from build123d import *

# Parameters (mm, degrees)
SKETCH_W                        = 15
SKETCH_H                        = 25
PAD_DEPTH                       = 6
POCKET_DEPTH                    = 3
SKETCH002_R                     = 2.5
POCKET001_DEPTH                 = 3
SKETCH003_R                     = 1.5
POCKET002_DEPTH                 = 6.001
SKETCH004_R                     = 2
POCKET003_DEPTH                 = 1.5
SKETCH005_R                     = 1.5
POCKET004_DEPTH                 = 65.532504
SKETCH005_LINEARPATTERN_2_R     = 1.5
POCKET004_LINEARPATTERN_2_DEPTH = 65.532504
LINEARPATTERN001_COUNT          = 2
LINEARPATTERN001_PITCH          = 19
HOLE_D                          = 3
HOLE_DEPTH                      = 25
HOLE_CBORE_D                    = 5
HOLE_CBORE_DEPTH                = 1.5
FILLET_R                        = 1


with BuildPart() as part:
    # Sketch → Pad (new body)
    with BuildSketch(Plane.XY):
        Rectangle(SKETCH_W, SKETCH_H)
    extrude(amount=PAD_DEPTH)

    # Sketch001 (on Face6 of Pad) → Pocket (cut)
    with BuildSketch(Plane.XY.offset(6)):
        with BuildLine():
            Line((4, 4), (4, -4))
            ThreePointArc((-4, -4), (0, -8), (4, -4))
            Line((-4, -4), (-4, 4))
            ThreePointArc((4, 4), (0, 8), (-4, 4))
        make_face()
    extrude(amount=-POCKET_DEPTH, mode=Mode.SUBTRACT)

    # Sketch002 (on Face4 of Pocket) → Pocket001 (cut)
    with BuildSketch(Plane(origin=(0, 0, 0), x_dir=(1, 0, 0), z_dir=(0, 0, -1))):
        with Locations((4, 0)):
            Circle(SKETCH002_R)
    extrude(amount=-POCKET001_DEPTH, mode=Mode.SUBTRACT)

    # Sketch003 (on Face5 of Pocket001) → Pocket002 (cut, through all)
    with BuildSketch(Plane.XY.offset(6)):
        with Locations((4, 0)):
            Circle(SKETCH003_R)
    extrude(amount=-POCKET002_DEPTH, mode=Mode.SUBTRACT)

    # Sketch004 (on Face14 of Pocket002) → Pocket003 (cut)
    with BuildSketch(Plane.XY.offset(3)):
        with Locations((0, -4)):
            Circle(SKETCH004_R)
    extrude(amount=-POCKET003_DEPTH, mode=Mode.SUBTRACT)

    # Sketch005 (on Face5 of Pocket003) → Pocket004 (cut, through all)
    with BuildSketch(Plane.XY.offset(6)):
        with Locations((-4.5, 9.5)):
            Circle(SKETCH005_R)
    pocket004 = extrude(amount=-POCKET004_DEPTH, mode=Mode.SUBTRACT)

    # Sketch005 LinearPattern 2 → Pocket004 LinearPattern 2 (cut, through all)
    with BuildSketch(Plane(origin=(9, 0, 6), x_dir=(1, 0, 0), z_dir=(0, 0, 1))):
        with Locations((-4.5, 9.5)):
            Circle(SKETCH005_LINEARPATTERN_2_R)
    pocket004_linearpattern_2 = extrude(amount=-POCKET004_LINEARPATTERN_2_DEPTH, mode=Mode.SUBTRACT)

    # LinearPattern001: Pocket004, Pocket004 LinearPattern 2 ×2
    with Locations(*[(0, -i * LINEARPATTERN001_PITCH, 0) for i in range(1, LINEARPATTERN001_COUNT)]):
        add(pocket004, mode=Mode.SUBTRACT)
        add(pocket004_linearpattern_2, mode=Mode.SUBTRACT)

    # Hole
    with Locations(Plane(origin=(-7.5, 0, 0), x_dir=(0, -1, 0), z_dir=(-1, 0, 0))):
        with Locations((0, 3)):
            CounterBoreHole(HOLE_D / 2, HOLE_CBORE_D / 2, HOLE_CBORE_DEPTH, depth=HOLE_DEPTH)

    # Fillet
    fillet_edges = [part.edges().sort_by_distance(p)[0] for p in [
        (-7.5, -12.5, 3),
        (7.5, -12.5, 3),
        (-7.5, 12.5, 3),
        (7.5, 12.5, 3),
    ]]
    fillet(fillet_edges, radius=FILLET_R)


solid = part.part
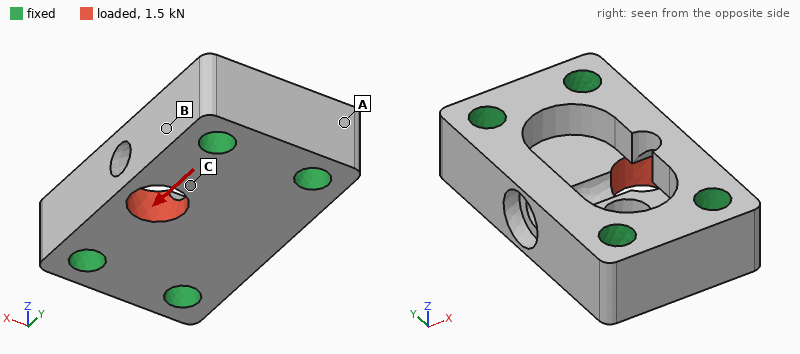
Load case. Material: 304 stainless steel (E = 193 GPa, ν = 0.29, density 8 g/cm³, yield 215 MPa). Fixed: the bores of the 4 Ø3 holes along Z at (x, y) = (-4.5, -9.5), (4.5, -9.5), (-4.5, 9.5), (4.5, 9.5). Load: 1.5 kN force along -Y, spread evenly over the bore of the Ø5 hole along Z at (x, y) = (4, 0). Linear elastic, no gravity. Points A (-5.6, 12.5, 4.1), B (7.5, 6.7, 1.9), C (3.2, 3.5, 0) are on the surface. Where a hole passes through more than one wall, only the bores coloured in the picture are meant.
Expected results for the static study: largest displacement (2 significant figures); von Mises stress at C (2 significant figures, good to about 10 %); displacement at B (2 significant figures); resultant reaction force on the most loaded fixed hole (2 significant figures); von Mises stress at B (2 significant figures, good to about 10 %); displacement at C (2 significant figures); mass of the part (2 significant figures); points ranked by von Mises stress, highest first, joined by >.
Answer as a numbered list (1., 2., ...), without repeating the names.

1. 1.5 µm
2. 40 MPa
3. 0.38 µm
4. 610 N
5. 19 MPa
6. 0.90 µm
7. 13 g
8. C > B > A
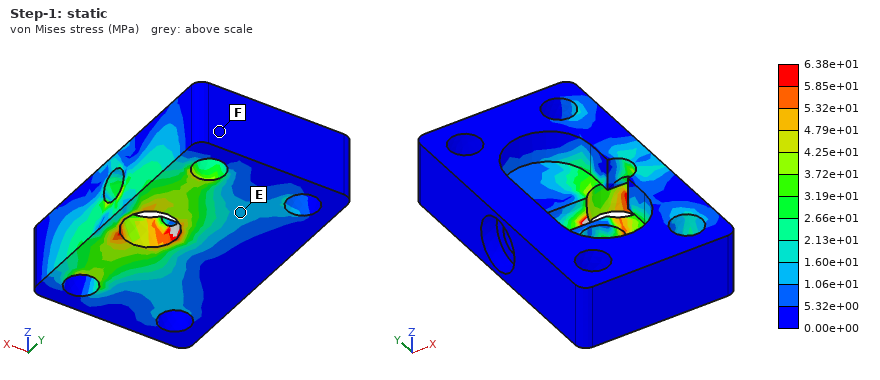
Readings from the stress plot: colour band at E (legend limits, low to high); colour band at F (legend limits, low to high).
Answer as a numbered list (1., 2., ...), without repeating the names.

1. 1.06e+01 to 1.60e+01 MPa
2. 0.00e+00 to 5.32e+00 MPa
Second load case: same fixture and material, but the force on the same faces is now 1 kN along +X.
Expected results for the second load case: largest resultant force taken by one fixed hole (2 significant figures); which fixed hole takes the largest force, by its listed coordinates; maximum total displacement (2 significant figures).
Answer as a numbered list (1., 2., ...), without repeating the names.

1. 340 N
2. (-4.5, 9.5)
3. 3.9 µm
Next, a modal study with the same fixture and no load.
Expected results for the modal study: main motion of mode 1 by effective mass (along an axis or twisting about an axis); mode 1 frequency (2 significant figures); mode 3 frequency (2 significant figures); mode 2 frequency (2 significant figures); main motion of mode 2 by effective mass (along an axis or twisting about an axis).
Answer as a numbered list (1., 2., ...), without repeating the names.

1. along Z
2. 66 kHz
3. 80 kHz
4. 73 kHz
5. along X
